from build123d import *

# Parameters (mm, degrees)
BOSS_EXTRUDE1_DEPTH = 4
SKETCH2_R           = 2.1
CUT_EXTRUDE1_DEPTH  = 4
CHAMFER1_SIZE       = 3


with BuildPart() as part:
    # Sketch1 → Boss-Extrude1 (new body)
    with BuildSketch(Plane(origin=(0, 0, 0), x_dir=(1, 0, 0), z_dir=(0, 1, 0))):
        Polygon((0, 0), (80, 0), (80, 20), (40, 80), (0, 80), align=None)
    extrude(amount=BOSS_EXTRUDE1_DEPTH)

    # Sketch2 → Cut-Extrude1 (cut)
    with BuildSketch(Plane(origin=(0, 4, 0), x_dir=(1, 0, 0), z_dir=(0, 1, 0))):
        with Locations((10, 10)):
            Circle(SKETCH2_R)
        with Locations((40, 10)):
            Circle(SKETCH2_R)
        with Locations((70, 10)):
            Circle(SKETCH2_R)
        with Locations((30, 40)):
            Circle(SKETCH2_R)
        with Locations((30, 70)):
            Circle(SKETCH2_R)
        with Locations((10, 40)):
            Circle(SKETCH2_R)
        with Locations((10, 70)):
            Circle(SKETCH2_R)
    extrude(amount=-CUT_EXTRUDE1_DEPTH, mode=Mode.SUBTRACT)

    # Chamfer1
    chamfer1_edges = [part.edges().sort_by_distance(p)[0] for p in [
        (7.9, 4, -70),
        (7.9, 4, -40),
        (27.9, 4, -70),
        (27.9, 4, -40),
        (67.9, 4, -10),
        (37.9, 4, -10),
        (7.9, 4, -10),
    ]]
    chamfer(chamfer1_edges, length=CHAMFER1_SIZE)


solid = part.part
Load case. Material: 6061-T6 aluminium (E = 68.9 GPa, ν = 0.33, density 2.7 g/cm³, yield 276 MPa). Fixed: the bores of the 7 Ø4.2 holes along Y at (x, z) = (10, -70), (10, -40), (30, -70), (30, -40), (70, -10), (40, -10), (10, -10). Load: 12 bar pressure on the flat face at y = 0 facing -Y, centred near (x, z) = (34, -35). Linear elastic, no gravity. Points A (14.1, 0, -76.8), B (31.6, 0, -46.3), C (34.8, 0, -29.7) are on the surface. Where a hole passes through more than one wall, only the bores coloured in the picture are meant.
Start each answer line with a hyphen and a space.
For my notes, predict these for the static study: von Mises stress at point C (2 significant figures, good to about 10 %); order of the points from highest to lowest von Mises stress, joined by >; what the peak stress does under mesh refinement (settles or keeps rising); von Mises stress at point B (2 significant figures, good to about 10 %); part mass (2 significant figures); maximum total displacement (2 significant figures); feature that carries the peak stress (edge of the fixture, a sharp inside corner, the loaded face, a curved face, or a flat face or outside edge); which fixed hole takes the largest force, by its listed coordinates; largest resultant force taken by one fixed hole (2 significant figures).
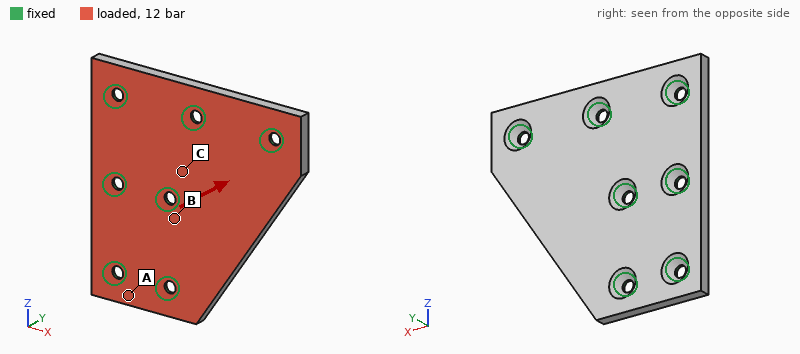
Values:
- 56 MPa
- B > C > A
- keeps rising
- 82 MPa
- 53 g
- 0.28 mm
- edge of the fixture
- (30, -40)
- 1.8 kN
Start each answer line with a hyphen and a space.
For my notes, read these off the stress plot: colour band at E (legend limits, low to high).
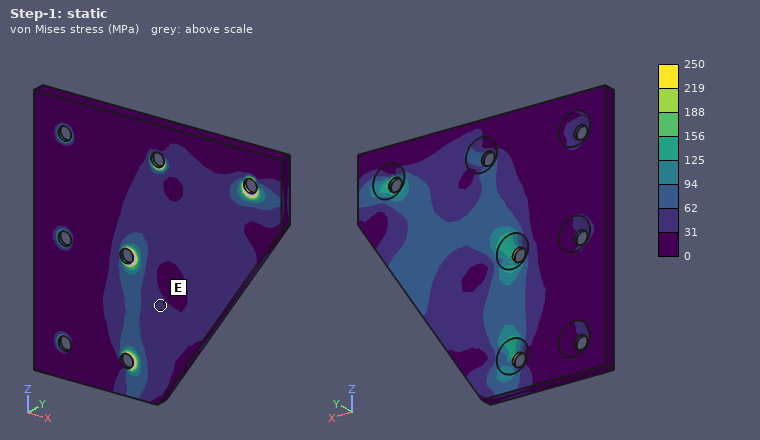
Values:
- 31 to 62 MPa
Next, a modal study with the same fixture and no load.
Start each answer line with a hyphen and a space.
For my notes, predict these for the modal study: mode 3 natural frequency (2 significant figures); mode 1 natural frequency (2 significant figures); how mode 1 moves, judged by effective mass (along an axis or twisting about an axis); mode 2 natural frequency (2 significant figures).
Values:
- 12 kHz
- 4200 Hz
- along Y
- 8600 Hz
